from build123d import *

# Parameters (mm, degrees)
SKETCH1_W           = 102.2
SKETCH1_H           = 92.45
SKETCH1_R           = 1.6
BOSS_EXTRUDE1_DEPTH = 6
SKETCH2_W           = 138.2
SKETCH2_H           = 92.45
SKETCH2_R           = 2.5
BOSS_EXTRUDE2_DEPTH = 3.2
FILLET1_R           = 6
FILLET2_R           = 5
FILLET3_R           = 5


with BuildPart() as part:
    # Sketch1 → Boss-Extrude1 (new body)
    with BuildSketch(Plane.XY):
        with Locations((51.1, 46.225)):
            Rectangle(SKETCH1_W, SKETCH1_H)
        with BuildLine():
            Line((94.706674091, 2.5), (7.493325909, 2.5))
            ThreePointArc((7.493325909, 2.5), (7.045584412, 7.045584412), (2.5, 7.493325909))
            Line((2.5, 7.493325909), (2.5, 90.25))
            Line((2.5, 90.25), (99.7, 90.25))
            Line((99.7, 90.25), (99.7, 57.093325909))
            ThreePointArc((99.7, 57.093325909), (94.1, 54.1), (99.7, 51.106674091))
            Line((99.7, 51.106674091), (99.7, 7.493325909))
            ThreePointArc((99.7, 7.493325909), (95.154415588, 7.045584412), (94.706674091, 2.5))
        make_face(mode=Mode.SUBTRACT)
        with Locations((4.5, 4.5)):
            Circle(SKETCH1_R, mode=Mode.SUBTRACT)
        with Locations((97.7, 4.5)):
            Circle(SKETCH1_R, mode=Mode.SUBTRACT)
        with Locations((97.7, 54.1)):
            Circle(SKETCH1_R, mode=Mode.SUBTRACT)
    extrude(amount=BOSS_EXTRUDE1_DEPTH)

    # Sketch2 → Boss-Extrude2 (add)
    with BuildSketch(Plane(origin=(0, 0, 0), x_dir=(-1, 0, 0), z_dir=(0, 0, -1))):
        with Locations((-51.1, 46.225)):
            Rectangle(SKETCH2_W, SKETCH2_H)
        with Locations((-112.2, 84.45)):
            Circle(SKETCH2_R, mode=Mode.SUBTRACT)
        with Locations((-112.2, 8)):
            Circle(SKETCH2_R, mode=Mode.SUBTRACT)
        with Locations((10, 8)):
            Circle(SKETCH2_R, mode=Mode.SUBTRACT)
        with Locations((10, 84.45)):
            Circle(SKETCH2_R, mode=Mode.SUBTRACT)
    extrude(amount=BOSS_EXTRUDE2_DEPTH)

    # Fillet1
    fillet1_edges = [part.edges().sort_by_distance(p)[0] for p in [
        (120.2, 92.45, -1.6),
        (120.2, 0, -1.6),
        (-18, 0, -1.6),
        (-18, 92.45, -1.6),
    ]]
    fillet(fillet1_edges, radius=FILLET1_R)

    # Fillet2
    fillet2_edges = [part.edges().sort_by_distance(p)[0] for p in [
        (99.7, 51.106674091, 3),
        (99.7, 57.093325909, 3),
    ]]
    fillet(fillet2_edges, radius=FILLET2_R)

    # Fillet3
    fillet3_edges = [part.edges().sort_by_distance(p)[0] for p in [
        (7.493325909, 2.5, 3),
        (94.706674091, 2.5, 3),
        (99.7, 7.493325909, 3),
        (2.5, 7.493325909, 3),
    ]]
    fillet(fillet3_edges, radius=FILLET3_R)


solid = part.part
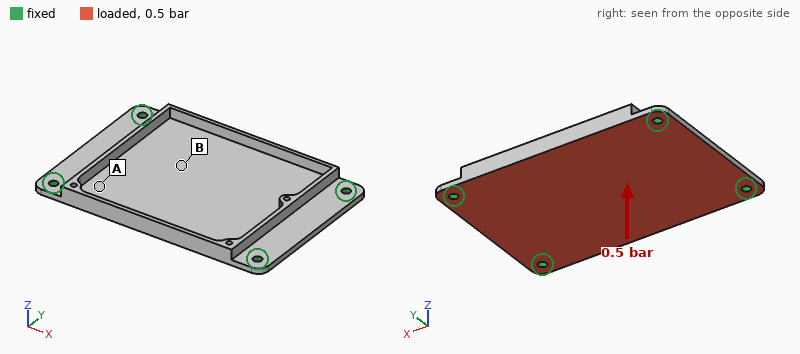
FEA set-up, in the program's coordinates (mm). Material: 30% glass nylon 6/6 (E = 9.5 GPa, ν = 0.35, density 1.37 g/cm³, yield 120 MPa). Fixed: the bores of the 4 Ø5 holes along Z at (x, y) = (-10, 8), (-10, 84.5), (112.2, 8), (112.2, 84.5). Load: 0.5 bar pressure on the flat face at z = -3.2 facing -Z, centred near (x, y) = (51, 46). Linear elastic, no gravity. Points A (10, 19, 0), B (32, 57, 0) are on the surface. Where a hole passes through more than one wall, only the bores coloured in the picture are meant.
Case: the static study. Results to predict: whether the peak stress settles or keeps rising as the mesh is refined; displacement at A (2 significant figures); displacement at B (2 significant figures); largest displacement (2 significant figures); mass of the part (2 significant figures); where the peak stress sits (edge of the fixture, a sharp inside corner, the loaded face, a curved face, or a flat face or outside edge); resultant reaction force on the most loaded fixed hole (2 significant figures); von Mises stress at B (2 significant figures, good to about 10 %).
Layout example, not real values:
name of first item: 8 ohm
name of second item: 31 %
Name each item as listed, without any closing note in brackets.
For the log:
whether the peak stress settles or keeps rising as the mesh is refined: keeps rising
displacement at A: 0.33 mm
displacement at B: 0.81 mm
largest displacement: 0.94 mm
mass of the part: 64 g
where the peak stress sits: edge of the fixture
resultant reaction force on the most loaded fixed hole: 210 N
von Mises stress at B: 11 MPa
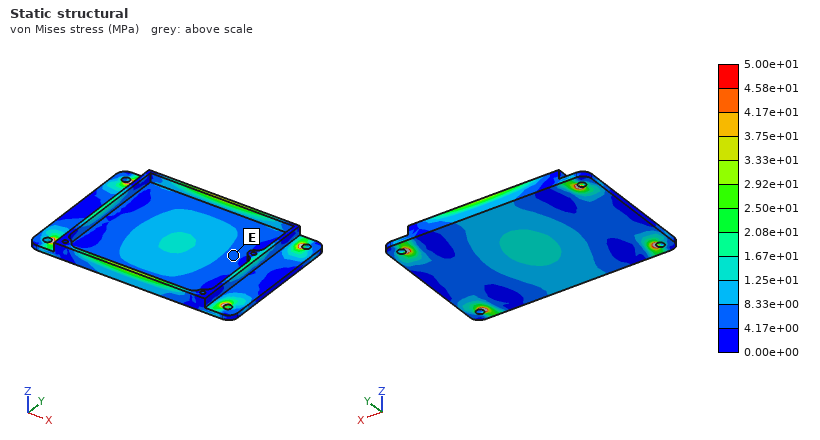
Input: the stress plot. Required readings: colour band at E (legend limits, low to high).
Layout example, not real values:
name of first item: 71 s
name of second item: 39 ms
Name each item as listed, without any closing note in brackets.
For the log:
colour band at E: 4.17e+00 to 8.33e+00 MPa
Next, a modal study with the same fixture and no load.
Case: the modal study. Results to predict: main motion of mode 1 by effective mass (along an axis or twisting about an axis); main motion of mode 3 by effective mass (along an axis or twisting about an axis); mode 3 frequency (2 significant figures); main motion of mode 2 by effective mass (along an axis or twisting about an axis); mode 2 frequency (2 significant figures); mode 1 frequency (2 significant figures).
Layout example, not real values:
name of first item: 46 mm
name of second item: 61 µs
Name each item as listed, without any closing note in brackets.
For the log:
main motion of mode 1 by effective mass: along Z
main motion of mode 3 by effective mass: twisting about Y
mode 3 frequency: 1500 Hz
main motion of mode 2 by effective mass: twisting about X
mode 2 frequency: 1000 Hz
mode 1 frequency: 640 Hz
